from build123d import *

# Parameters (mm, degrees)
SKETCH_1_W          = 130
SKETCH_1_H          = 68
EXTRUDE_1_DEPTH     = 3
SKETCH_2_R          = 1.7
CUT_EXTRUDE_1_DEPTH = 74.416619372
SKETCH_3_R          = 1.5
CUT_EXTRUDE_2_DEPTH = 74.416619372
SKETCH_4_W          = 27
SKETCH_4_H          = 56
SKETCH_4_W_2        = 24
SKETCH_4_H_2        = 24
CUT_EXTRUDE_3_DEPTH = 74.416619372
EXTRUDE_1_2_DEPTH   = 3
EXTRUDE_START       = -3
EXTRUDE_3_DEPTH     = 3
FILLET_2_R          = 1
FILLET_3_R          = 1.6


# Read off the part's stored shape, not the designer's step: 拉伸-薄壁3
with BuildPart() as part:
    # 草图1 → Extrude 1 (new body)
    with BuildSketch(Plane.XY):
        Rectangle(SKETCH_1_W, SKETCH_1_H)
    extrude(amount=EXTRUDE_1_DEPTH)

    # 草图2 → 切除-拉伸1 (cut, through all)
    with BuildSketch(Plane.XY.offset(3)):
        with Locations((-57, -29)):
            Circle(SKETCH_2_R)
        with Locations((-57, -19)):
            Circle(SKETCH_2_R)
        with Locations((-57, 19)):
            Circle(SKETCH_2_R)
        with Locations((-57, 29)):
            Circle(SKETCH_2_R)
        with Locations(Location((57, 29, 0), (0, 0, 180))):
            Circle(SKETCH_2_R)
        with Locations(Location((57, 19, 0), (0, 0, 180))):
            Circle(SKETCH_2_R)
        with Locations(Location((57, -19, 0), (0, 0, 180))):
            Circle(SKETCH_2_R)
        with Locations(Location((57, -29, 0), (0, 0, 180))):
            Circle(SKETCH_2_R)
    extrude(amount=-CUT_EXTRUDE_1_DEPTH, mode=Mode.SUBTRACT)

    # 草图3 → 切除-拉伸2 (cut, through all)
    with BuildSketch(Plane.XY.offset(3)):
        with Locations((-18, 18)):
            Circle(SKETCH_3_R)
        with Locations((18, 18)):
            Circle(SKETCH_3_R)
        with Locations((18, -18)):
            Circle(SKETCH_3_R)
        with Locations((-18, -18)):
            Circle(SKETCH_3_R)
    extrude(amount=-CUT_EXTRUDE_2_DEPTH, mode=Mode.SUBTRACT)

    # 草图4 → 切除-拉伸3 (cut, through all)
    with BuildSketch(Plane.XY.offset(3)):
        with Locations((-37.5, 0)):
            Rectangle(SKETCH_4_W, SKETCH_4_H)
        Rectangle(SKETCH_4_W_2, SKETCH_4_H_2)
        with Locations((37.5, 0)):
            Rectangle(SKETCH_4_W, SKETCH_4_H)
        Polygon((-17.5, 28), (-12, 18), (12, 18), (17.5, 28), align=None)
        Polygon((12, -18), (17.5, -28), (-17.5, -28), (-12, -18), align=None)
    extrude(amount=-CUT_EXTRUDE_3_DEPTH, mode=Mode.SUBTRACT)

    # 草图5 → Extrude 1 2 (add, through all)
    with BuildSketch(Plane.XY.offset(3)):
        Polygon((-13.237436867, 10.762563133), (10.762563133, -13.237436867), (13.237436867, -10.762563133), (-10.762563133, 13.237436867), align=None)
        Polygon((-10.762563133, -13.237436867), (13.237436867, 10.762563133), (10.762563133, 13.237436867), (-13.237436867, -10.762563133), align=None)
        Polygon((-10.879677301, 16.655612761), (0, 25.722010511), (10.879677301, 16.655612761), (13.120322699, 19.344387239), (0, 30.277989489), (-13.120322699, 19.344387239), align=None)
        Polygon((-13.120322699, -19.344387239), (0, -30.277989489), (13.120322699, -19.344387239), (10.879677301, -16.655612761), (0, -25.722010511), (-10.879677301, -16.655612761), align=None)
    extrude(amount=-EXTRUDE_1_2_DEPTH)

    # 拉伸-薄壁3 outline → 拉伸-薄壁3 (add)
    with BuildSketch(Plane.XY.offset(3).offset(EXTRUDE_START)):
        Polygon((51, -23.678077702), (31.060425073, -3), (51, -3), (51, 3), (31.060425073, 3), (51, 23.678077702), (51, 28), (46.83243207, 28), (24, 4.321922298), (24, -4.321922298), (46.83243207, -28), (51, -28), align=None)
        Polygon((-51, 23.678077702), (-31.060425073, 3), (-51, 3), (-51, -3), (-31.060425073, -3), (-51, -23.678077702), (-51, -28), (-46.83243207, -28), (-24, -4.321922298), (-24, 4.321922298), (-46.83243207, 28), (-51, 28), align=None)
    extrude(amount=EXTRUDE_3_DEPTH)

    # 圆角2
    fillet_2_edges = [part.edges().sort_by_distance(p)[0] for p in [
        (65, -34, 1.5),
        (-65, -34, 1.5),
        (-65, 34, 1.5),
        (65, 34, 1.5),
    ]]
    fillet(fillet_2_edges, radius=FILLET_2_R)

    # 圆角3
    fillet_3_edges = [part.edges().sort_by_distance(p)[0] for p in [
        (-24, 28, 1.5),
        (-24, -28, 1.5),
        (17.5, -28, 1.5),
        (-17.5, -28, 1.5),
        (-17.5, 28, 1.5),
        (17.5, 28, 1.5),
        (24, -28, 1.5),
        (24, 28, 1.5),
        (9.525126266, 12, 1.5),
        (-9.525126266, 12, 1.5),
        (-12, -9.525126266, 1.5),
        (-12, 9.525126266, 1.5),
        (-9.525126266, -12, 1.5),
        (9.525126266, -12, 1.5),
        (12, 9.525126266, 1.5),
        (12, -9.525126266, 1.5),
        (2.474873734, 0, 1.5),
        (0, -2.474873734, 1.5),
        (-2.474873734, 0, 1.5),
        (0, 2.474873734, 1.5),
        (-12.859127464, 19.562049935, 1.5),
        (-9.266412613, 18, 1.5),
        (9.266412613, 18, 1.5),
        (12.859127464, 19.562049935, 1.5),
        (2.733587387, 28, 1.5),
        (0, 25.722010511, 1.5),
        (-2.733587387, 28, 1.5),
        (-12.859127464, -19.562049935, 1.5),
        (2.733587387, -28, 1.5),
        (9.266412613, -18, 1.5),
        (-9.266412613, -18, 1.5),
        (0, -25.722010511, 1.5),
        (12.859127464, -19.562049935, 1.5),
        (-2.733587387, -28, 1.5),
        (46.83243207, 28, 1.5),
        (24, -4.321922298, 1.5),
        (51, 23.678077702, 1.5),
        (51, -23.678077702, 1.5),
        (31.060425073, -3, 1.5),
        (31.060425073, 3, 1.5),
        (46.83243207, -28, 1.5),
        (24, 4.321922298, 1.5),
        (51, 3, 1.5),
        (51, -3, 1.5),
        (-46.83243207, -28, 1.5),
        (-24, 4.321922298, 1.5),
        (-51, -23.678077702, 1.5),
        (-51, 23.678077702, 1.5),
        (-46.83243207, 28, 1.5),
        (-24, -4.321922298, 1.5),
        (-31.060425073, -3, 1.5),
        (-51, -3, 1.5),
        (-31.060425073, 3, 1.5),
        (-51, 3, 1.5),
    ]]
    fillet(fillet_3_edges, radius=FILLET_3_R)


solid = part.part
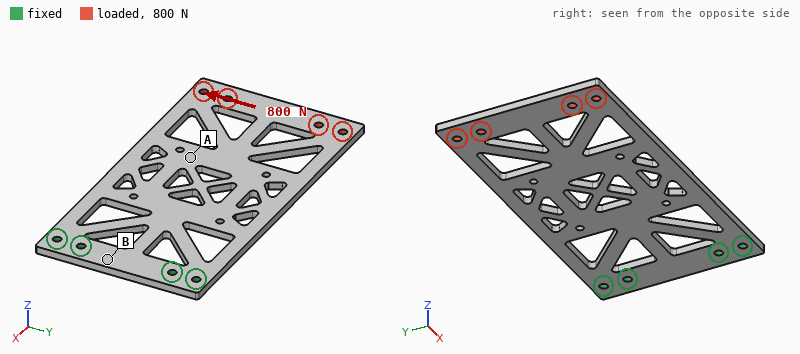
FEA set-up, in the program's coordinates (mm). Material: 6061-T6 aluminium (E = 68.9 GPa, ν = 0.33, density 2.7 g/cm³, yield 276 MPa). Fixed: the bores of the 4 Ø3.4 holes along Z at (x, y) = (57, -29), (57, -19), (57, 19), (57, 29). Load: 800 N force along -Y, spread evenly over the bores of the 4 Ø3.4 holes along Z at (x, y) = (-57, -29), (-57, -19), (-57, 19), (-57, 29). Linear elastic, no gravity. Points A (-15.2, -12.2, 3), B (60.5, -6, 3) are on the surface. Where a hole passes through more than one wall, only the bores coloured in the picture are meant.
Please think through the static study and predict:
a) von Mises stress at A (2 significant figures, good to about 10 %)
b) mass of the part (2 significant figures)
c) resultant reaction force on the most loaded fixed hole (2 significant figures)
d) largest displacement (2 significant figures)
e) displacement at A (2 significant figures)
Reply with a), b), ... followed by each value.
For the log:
a) 17 MPa
b) 50 g
c) 1.6 kN
d) 0.22 mm
e) 0.10 mm
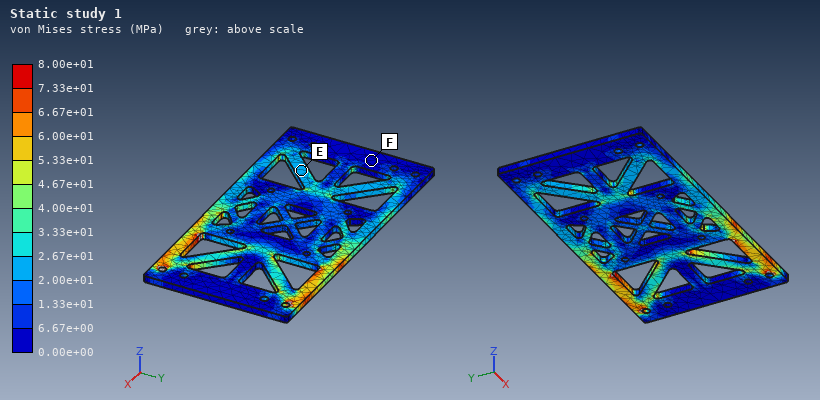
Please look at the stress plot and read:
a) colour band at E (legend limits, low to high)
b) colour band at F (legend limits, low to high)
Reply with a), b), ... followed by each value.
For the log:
a) 2.00e+01 to 2.67e+01 MPa
b) 0.00e+00 to 6.67e+00 MPa
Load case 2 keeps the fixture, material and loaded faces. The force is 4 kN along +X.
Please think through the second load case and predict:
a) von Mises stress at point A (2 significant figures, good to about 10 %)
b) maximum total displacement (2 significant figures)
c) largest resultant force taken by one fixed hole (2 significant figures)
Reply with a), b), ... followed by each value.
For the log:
a) 26 MPa
b) 0.10 mm
c) 1.5 kN
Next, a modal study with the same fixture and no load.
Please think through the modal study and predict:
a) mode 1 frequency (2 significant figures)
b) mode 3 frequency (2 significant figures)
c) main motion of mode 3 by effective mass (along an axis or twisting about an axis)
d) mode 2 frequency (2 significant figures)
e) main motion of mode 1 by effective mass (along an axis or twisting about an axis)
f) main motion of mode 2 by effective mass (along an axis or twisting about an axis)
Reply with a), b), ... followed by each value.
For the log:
a) 130 Hz
b) 840 Hz
c) along Z
d) 550 Hz
e) along Z
f) twisting about X
